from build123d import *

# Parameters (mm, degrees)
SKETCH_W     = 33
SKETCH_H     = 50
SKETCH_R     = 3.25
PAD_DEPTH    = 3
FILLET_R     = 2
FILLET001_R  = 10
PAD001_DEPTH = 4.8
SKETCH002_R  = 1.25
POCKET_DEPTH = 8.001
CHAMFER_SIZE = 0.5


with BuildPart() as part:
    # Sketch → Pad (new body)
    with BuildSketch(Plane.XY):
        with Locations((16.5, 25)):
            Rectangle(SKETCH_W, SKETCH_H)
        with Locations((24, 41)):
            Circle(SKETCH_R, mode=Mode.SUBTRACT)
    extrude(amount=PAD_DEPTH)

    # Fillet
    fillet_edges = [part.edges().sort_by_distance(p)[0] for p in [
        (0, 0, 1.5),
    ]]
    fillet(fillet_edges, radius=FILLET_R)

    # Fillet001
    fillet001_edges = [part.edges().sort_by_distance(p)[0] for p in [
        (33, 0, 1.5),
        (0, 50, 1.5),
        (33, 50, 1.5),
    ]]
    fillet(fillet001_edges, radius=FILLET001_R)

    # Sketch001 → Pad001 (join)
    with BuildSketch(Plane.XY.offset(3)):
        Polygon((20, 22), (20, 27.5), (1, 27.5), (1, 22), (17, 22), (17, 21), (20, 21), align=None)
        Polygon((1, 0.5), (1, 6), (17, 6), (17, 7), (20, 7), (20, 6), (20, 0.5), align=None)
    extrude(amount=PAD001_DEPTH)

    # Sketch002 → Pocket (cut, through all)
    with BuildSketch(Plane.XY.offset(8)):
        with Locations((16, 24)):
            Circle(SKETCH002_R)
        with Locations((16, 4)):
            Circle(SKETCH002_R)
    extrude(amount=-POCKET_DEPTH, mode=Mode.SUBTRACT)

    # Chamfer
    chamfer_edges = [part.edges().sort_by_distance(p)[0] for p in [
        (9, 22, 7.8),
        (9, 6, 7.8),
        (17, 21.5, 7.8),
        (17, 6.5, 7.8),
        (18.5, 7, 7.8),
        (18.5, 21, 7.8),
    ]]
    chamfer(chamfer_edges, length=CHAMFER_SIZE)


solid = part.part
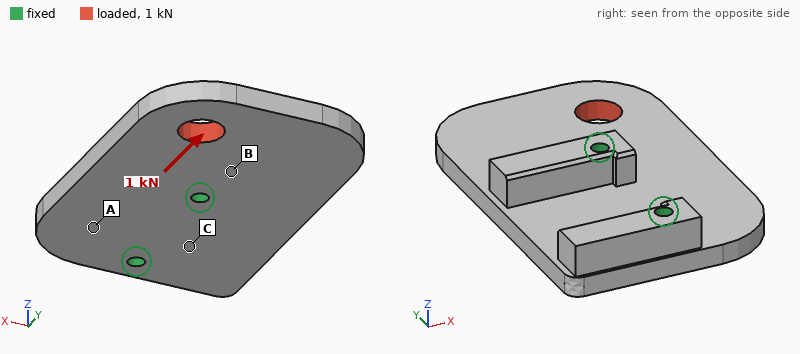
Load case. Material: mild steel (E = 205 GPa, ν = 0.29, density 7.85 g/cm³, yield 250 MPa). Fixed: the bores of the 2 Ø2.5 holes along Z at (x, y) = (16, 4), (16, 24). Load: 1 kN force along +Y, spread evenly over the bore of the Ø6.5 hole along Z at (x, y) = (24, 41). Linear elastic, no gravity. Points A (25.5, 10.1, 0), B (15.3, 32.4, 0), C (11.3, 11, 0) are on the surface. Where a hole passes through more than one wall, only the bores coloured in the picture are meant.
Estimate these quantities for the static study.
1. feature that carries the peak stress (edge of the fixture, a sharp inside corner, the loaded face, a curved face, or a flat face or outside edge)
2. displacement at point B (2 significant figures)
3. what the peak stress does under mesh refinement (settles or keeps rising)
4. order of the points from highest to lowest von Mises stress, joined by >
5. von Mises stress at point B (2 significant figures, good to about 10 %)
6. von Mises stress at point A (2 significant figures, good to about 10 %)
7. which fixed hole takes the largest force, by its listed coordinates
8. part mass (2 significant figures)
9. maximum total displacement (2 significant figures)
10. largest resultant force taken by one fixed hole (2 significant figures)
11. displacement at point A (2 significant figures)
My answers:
edge of the fixture
1.3 µm
keeps rising
B > A > C
16 MPa
11 MPa
(16, 24)
44 g
5.2 µm
830 N
0.93 µm
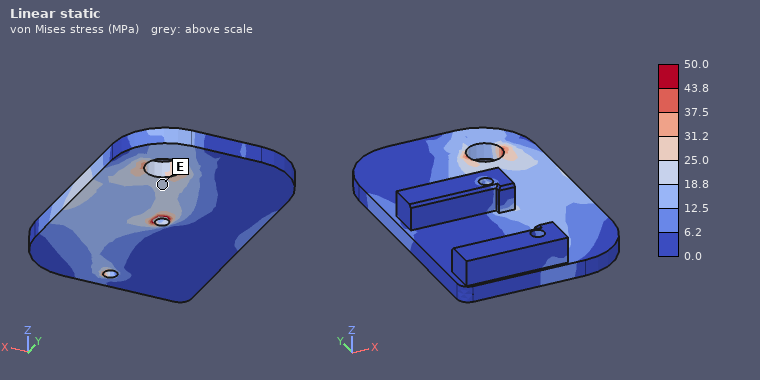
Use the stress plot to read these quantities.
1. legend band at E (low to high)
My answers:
18.8 to 25.0 MPa
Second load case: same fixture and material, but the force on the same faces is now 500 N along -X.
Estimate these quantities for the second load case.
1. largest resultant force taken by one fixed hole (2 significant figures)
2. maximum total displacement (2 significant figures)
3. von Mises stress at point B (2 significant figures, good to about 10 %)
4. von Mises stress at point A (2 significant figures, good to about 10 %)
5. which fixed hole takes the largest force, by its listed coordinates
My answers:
850 N
5.6 µm
12 MPa
7.1 MPa
(16, 24)
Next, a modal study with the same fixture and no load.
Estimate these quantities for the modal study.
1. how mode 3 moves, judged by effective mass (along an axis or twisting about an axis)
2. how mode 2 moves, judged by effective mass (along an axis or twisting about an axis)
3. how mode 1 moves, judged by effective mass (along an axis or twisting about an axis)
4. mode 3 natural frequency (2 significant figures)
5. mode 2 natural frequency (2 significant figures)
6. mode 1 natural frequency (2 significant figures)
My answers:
along Z
twisting about Y
along Z
11 kHz
7100 Hz
4200 Hz
